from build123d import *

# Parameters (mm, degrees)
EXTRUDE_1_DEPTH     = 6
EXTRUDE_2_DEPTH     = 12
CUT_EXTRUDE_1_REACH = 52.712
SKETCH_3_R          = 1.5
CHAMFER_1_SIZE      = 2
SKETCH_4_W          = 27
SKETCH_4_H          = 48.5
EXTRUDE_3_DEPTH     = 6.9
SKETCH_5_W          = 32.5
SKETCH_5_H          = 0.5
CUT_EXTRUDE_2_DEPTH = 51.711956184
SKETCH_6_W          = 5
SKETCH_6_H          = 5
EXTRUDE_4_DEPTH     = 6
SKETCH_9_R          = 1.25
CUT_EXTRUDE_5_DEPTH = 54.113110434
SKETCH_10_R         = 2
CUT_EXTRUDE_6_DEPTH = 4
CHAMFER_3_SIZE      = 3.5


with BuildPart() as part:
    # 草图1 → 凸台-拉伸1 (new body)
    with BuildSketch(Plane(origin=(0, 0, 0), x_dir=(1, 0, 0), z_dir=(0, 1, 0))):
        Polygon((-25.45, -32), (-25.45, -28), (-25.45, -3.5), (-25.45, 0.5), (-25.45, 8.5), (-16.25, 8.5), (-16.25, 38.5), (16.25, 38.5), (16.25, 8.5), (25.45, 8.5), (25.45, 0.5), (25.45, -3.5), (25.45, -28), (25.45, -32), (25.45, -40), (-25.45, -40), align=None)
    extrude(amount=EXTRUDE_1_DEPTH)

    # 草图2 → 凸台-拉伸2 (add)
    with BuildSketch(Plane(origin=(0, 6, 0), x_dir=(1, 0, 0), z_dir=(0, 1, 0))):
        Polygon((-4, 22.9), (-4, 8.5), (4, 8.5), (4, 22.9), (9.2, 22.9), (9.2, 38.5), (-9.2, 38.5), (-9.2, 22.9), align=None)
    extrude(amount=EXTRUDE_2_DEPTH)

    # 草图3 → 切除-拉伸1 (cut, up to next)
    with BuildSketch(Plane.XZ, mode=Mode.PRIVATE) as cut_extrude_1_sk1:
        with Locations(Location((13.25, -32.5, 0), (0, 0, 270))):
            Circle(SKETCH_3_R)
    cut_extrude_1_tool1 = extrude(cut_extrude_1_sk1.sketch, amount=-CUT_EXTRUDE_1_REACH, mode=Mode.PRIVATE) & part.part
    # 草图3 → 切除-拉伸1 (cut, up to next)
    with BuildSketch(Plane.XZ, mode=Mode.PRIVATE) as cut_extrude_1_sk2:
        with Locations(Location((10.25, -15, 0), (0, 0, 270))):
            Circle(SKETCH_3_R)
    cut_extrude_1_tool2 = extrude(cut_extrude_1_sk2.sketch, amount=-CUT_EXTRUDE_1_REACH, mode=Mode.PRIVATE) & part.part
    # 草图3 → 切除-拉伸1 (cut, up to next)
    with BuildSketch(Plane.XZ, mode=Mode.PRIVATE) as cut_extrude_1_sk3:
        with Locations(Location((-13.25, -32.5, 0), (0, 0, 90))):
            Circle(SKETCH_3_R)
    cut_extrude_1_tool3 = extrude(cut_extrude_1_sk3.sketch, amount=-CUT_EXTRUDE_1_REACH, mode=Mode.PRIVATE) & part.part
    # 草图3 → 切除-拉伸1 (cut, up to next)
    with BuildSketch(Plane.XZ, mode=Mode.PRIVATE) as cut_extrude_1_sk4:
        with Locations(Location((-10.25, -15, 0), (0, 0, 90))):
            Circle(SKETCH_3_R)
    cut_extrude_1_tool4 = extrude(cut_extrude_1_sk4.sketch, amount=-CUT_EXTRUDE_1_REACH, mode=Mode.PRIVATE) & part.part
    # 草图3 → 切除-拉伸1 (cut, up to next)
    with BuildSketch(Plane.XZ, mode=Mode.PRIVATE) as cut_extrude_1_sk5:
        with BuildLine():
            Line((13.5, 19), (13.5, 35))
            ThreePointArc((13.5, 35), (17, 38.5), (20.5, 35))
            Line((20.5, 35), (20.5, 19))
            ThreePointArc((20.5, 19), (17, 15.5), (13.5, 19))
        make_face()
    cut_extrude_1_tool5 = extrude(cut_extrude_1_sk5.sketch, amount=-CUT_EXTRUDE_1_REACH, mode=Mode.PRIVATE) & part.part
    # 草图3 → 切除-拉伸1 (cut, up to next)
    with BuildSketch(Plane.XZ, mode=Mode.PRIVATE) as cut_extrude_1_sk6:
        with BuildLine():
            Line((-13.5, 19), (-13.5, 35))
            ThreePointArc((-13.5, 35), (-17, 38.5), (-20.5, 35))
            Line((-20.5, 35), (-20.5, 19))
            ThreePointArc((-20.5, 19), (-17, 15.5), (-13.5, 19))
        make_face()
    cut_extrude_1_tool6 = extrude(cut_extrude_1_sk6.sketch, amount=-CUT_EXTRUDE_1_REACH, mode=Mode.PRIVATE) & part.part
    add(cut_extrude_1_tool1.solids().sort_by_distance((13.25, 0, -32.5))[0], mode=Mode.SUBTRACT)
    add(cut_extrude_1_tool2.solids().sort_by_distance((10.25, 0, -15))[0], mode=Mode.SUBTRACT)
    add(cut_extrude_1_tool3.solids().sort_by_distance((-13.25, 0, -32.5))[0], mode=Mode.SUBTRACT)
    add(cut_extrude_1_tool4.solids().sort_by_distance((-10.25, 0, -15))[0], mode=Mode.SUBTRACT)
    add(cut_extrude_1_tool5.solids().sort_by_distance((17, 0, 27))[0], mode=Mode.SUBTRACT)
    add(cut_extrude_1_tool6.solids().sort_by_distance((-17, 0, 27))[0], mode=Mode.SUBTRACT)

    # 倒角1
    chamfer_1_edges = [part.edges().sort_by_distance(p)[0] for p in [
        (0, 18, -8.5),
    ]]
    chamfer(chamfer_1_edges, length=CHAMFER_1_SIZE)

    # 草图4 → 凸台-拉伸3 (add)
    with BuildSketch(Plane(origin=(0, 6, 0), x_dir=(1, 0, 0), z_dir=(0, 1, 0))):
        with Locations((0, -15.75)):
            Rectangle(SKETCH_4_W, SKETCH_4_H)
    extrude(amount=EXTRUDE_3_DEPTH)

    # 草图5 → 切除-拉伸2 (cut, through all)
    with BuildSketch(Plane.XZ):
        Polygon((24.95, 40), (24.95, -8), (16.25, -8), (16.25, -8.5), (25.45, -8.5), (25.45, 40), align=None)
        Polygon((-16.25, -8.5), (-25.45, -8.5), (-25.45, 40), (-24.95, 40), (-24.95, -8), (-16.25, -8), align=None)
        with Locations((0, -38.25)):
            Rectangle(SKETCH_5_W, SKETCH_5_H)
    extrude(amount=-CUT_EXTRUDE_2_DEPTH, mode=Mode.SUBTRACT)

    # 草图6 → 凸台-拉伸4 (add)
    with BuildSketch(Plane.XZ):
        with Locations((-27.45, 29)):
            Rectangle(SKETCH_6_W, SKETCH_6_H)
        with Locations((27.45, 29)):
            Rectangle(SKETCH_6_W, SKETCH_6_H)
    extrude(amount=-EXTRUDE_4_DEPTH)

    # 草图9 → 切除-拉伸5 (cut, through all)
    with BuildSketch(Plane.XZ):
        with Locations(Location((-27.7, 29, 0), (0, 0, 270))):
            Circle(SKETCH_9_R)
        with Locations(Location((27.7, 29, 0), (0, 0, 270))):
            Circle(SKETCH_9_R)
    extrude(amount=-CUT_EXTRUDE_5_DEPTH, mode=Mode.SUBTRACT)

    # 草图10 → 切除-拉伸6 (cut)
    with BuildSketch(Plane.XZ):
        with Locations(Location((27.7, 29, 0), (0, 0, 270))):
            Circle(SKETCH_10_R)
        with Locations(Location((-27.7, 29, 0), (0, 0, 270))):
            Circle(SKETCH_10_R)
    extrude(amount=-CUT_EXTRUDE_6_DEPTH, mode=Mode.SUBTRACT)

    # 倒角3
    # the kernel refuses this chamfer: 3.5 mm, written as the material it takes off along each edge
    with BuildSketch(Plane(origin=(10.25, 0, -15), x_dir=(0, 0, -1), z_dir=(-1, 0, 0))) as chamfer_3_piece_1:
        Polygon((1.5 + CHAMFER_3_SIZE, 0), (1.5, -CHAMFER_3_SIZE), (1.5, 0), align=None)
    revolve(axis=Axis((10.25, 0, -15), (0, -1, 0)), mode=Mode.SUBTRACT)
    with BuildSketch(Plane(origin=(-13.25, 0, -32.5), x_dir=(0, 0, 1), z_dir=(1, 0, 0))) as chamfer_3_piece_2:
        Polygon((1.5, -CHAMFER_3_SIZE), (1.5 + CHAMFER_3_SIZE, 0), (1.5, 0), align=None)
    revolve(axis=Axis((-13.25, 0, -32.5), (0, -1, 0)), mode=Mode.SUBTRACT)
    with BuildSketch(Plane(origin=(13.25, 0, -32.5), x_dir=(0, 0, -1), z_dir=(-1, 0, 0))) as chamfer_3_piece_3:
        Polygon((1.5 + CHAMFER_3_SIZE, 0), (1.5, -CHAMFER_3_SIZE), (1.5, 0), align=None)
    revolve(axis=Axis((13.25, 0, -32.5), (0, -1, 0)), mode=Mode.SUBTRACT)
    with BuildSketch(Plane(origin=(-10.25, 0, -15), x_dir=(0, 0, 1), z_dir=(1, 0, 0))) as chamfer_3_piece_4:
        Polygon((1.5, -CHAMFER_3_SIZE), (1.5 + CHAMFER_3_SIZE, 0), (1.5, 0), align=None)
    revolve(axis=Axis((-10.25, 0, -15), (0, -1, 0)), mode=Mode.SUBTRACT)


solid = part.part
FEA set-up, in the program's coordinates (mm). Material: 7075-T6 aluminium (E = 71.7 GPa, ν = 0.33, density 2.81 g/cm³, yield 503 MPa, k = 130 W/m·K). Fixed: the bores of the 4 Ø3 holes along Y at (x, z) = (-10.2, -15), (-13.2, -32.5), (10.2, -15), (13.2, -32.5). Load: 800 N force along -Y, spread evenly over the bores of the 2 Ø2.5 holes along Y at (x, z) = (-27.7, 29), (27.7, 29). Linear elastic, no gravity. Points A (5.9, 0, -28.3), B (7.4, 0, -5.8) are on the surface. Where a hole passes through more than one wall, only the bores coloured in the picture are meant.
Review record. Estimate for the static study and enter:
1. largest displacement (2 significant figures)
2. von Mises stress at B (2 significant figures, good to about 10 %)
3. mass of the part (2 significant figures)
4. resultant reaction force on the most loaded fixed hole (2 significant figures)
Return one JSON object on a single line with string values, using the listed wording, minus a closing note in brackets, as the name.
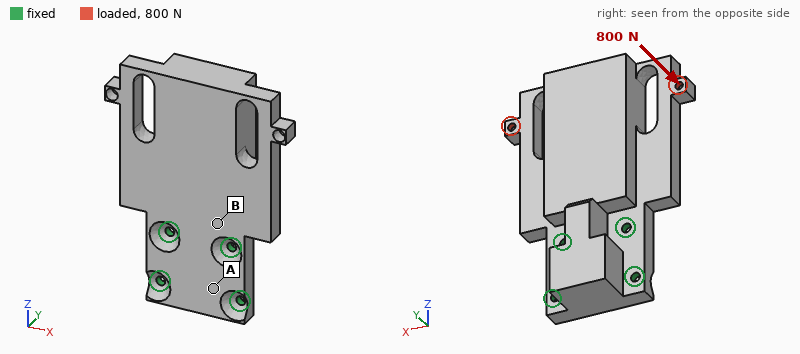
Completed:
{"largest displacement": "0.31 mm", "von Mises stress at B": "39 MPa", "mass of the part": "89 g", "resultant reaction force on the most loaded fixed hole": "1.3 kN"}
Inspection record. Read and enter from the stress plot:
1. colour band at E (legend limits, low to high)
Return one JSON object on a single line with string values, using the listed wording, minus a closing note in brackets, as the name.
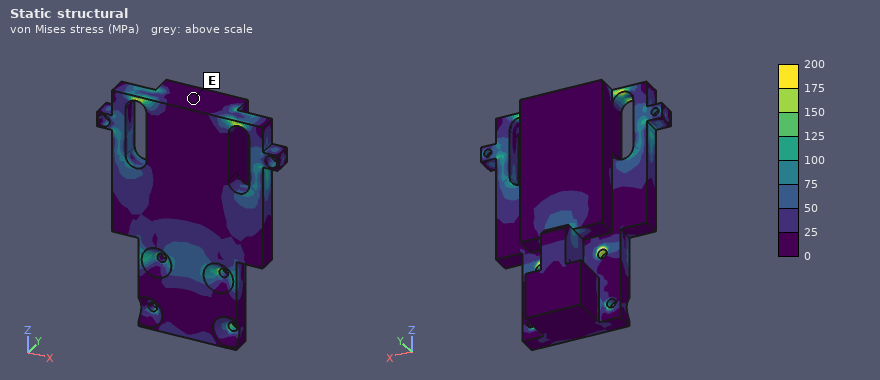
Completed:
{"colour band at E": "0 to 25 MPa"}
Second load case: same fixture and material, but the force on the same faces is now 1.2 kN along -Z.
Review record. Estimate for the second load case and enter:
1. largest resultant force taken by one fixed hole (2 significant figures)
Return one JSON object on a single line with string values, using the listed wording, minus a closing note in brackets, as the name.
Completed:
{"largest resultant force taken by one fixed hole": "460 N"}
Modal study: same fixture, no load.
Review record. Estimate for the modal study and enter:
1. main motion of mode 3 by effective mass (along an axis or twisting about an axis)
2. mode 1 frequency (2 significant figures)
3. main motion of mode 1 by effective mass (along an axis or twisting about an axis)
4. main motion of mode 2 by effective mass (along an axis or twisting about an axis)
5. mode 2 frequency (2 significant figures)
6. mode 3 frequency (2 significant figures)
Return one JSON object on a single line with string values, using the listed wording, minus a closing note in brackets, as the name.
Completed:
{"main motion of mode 3 by effective mass": "twisting about Z", "mode 1 frequency": "1800 Hz", "main motion of mode 1 by effective mass": "along Y", "main motion of mode 2 by effective mass": "along X", "mode 2 frequency": "4500 Hz", "mode 3 frequency": "5200 Hz"}
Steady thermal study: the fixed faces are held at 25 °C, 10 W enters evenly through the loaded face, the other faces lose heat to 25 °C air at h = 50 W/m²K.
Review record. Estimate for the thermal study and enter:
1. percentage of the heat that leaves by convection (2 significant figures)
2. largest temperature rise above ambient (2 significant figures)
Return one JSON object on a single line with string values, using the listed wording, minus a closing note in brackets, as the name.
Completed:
{"percentage of the heat that leaves by convection": "29 %", "largest temperature rise above ambient": "31 K"}
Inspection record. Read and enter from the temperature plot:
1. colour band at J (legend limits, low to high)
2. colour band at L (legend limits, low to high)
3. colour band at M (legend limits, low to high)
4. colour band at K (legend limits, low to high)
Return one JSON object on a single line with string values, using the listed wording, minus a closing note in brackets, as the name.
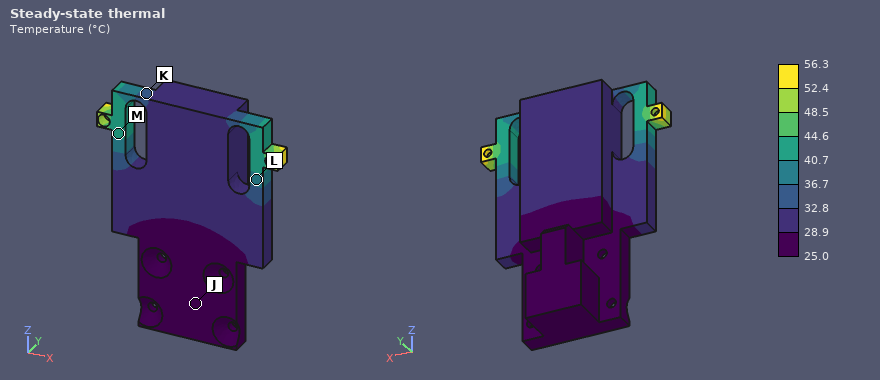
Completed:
{"colour band at J": "25.0 to 28.9 °C", "colour band at L": "36.7 to 40.7 °C", "colour band at M": "40.7 to 44.6 °C", "colour band at K": "32.8 to 36.7 °C"}
